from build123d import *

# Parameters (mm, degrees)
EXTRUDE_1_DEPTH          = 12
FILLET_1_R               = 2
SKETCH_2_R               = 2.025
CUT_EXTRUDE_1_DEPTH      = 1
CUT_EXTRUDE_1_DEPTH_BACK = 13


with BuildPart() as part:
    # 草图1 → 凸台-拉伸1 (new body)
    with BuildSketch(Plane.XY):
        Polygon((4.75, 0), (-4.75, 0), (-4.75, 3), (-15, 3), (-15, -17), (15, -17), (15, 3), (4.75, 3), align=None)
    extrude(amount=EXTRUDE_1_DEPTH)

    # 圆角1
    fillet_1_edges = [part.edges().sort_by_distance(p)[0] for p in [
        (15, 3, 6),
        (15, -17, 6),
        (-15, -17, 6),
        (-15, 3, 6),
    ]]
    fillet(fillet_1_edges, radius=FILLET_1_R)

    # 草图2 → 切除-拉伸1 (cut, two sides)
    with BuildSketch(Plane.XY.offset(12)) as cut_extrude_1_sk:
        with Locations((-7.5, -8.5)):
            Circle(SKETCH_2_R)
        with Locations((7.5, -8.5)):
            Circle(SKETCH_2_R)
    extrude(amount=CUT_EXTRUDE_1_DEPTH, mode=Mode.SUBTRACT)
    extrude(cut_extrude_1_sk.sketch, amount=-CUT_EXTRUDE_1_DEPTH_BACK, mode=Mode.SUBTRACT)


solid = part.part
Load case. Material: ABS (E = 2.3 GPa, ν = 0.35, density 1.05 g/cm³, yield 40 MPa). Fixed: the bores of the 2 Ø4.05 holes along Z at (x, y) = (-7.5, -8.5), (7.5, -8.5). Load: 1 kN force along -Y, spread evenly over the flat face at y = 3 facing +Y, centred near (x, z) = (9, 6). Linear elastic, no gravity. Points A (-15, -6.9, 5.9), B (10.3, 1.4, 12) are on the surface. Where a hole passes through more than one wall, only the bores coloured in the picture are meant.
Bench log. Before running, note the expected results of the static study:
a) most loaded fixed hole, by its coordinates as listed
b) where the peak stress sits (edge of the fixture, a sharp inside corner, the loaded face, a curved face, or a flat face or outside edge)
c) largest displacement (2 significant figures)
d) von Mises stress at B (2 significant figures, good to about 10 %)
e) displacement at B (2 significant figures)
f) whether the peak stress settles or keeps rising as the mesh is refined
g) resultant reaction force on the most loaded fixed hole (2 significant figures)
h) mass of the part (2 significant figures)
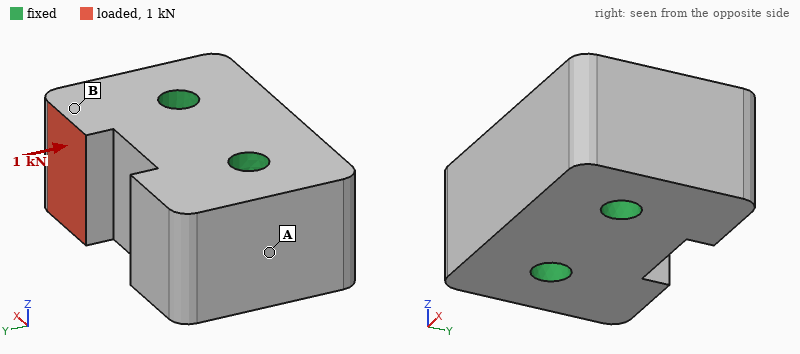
(7.5, -8.5)
edge of the fixture
57 µm
10 MPa
50 µm
keeps rising
1.0 kN
6.8 g
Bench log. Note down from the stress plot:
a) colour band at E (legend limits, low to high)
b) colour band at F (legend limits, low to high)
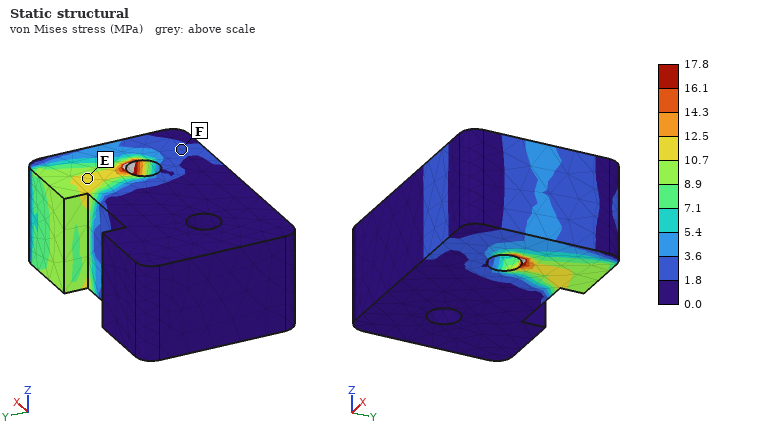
10.7 to 12.5 MPa
1.8 to 3.6 MPa
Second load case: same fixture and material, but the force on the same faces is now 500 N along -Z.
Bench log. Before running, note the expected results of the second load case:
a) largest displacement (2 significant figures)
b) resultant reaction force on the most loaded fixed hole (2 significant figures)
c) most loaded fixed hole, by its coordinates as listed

0.13 mm
460 N
(7.5, -8.5)
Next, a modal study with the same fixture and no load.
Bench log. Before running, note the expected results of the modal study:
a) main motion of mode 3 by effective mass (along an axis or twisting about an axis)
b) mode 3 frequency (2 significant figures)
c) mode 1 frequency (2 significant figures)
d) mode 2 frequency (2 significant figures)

twisting about Y
15 kHz
14 kHz
14 kHz
